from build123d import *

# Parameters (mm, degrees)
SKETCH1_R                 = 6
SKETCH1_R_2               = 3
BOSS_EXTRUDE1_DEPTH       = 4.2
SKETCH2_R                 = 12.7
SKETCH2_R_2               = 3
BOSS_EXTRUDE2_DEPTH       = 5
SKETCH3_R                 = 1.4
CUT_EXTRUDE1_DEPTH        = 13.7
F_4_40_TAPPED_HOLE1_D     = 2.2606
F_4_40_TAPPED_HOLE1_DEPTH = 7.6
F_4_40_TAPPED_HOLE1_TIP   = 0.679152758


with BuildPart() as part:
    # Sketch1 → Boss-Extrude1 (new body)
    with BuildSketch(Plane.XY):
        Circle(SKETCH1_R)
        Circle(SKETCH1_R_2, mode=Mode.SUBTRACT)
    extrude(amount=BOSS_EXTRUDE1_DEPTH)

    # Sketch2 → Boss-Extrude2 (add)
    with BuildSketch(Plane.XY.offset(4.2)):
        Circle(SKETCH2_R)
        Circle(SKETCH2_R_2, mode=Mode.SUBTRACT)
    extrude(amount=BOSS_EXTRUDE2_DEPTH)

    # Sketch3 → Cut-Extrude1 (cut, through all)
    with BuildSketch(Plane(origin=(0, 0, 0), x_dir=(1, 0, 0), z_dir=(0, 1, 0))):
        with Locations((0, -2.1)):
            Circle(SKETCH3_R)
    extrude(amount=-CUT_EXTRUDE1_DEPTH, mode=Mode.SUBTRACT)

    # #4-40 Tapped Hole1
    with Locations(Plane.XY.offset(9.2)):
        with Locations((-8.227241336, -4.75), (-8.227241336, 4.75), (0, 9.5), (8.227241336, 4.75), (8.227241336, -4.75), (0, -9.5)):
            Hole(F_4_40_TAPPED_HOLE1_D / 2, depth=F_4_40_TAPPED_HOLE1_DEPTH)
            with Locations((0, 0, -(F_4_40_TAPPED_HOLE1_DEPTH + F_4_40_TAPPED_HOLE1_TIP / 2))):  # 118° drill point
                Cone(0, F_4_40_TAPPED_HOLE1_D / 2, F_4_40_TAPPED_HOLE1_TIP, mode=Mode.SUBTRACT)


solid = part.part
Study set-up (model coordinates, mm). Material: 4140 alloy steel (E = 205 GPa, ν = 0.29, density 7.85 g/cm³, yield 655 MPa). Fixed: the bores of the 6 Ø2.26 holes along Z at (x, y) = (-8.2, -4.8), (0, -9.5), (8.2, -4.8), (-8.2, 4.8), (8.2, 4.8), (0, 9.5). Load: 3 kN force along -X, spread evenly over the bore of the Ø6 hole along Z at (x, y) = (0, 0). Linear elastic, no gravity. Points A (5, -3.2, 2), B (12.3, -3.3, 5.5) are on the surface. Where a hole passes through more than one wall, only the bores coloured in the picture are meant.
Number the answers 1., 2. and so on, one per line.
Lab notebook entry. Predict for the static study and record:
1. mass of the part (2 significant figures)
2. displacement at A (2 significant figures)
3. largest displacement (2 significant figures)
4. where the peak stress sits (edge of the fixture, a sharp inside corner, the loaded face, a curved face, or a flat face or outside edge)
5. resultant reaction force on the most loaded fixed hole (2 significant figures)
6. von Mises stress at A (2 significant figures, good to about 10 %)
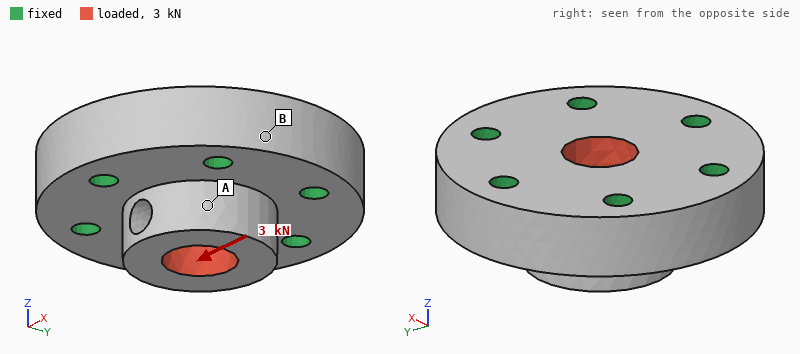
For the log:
1. 20 g
2. 1.5 µm
3. 2.4 µm
4. the loaded face
5. 710 N
6. 19 MPa
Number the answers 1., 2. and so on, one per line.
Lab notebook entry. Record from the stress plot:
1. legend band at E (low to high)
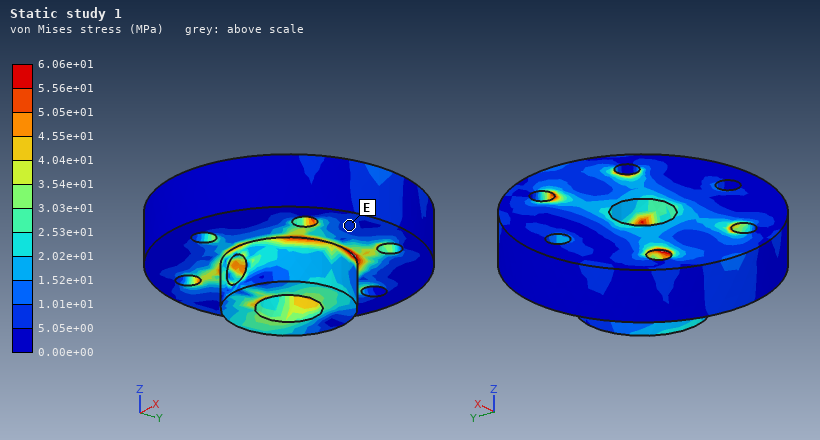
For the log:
1. 5.05e+00 to 1.01e+01 MPa
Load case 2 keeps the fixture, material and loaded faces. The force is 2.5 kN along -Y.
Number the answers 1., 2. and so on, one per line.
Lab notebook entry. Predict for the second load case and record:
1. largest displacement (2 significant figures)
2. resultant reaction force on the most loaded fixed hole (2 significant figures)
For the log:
1. 1.9 µm
2. 670 N
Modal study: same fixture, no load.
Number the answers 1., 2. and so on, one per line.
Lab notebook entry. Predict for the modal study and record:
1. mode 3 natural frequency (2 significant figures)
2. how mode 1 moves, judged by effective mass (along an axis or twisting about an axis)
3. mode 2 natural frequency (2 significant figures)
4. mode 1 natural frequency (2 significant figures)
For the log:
1. 92 kHz
2. along Z
3. 90 kHz
4. 84 kHz
